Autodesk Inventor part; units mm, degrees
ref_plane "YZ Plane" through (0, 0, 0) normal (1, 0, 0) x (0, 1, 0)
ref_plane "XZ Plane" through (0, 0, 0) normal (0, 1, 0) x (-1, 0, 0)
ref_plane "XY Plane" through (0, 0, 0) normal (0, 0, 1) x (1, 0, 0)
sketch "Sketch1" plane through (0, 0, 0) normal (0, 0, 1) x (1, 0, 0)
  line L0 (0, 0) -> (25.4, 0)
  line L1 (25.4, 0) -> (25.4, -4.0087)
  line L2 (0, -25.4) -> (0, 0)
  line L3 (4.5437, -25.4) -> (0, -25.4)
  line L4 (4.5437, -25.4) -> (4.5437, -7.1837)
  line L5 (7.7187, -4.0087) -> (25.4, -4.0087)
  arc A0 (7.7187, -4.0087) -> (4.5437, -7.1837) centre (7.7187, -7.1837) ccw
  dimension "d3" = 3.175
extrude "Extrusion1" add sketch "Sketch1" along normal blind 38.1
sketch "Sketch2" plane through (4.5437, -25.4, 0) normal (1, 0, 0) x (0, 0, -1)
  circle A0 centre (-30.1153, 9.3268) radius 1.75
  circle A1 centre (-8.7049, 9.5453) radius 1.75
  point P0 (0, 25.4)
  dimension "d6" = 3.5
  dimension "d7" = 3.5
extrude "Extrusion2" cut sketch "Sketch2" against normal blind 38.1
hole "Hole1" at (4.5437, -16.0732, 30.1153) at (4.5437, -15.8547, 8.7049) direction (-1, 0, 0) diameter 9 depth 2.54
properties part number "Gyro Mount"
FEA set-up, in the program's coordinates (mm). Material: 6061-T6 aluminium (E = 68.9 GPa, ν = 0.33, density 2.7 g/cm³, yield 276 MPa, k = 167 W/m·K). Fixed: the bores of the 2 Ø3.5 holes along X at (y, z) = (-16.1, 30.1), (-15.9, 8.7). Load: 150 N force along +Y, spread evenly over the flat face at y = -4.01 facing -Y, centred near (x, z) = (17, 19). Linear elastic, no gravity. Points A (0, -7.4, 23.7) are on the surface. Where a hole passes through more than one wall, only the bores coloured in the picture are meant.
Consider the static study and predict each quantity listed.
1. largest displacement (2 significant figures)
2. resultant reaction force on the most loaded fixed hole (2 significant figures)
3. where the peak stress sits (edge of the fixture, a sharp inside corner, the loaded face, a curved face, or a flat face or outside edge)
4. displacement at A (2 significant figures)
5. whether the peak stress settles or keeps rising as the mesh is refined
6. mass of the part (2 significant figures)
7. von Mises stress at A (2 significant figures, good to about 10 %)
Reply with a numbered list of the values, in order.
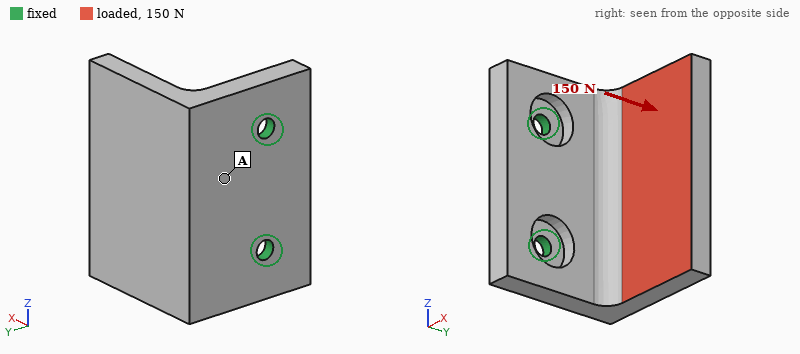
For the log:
1. 91 µm
2. 77 N
3. edge of the fixture
4. 17 µm
5. keeps rising
6. 20 g
7. 15 MPa
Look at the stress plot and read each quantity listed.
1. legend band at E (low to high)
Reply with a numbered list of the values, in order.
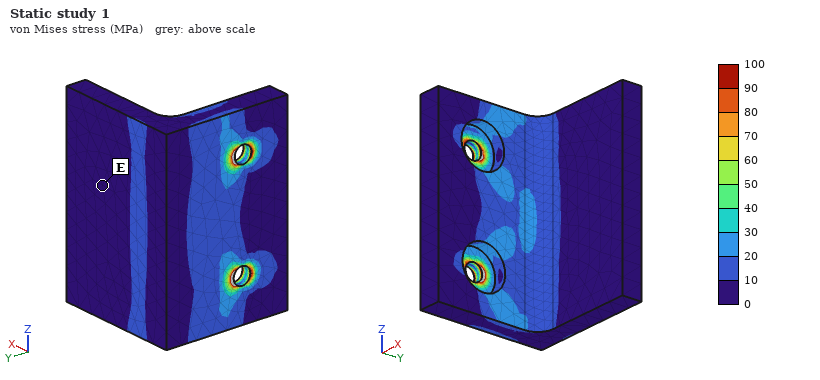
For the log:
1. 0 to 10 MPa
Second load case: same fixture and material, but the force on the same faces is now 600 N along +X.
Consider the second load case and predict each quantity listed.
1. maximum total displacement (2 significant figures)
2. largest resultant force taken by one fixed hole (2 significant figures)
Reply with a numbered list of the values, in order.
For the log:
1. 0.18 mm
2. 320 N
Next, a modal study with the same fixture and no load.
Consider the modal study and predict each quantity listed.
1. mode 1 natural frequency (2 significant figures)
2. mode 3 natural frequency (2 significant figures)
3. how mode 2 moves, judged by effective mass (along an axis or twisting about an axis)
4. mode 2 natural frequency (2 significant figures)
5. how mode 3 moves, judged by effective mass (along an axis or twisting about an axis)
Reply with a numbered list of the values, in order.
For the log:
1. 2400 Hz
2. 8800 Hz
3. along Z
4. 5300 Hz
5. along X
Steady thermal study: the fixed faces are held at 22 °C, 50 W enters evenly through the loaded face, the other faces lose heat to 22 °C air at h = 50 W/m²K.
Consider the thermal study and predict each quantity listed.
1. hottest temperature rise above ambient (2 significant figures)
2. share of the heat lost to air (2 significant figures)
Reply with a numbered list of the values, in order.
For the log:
1. 54 K
2. 9.6 %
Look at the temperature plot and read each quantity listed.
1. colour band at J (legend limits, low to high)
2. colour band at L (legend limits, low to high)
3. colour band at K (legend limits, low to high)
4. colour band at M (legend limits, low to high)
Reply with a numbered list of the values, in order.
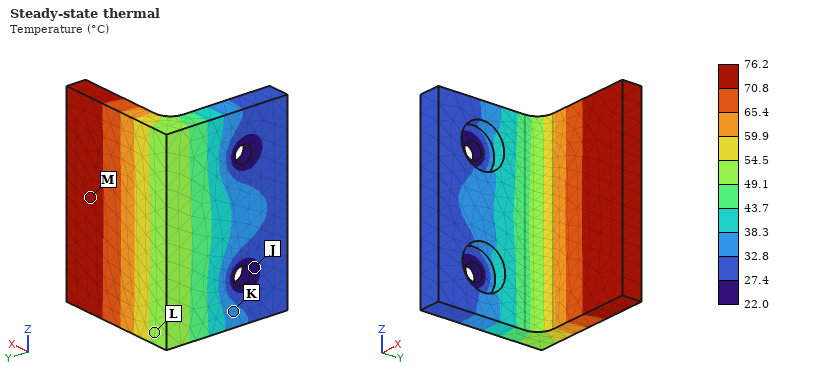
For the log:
1. 22.0 to 27.4 °C
2. 49.1 to 54.5 °C
3. 32.8 to 38.3 °C
4. 70.8 to 76.2 °C
